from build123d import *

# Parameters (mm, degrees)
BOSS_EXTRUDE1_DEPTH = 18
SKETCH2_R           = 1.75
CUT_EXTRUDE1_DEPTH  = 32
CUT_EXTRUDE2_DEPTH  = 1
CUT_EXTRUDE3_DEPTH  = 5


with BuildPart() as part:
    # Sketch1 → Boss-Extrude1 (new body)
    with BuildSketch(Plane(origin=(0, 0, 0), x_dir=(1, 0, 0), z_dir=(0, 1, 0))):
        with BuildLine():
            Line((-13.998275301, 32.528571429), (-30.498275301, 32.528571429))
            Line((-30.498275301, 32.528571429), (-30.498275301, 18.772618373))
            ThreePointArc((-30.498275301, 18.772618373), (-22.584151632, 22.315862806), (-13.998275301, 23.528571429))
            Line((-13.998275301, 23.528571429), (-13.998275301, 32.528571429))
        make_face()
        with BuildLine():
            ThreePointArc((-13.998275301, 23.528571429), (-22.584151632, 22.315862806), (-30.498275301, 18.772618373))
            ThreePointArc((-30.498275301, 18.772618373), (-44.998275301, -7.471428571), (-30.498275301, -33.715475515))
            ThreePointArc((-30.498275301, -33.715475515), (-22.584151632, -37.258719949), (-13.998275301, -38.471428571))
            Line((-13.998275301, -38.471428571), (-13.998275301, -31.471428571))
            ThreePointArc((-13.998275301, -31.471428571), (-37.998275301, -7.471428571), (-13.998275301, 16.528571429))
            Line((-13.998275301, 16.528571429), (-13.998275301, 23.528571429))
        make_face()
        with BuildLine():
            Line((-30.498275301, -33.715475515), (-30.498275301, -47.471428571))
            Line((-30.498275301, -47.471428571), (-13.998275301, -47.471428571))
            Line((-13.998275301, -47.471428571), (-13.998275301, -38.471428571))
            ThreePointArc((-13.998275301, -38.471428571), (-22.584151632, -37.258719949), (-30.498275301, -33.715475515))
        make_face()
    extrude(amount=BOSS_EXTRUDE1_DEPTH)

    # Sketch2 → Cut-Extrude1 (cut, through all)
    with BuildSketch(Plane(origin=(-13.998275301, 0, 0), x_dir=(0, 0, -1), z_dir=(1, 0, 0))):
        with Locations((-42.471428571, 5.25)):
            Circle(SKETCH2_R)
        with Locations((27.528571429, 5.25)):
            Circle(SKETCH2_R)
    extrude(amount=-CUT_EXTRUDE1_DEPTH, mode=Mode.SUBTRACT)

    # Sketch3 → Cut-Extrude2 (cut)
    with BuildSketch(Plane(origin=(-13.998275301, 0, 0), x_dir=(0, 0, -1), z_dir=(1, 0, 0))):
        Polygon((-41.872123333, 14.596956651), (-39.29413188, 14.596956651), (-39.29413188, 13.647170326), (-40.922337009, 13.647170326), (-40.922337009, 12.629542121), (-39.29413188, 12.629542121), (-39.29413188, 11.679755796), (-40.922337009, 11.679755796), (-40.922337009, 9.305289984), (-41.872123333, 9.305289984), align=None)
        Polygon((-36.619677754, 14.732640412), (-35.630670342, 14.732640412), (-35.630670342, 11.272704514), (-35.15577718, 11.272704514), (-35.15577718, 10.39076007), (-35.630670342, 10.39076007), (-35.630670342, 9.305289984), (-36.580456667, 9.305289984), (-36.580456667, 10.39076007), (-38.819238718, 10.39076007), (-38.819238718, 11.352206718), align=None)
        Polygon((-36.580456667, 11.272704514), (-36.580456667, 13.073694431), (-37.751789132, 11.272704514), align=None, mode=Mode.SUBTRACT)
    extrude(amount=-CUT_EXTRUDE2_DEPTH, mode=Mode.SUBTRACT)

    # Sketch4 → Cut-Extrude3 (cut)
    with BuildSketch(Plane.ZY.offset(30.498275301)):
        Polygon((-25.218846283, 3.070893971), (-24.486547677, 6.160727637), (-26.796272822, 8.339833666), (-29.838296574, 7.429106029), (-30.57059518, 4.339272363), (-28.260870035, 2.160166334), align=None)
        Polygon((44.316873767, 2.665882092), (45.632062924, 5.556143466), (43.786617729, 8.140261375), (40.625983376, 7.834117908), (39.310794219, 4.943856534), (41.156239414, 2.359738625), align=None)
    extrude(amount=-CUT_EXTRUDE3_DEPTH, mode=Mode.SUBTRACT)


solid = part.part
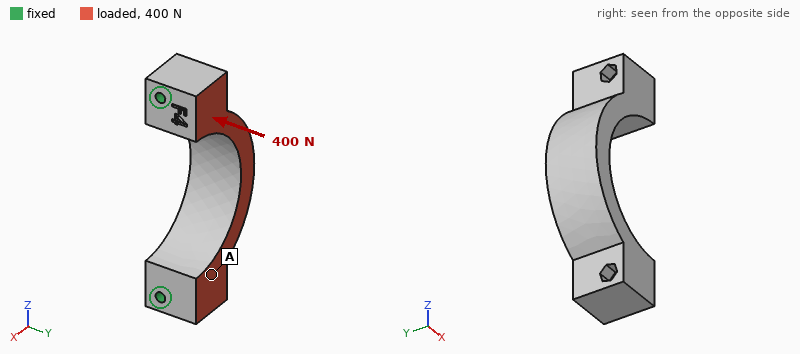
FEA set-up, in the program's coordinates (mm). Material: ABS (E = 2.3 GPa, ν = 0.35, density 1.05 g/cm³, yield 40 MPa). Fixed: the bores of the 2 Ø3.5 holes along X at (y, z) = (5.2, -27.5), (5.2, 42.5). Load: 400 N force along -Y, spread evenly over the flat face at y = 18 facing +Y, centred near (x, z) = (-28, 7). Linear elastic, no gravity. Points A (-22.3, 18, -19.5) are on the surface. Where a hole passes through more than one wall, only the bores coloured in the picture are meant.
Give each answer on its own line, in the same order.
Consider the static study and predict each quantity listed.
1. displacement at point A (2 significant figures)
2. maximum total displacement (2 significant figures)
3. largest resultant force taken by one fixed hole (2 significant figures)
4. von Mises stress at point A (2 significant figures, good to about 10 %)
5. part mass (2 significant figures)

0.076 mm
0.25 mm
200 N
2.3 MPa
17 g
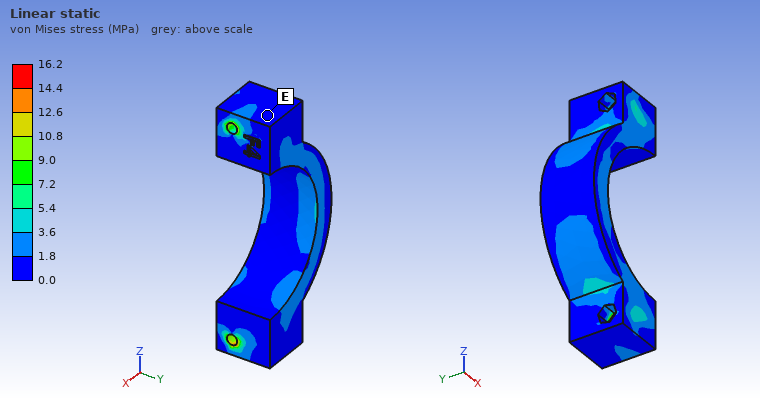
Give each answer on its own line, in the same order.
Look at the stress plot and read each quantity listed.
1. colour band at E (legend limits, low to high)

0.0 to 1.8 MPa
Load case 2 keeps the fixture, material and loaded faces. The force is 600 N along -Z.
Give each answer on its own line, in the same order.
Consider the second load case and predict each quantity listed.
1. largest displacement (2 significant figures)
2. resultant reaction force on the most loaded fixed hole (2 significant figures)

99 µm
310 N
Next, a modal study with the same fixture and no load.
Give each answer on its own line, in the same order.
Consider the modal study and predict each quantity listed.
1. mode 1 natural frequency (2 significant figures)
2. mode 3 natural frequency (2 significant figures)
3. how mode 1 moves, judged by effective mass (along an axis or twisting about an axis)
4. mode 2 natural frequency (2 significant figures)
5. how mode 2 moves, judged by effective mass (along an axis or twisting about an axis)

1900 Hz
5000 Hz
along Y
3800 Hz
along Z
